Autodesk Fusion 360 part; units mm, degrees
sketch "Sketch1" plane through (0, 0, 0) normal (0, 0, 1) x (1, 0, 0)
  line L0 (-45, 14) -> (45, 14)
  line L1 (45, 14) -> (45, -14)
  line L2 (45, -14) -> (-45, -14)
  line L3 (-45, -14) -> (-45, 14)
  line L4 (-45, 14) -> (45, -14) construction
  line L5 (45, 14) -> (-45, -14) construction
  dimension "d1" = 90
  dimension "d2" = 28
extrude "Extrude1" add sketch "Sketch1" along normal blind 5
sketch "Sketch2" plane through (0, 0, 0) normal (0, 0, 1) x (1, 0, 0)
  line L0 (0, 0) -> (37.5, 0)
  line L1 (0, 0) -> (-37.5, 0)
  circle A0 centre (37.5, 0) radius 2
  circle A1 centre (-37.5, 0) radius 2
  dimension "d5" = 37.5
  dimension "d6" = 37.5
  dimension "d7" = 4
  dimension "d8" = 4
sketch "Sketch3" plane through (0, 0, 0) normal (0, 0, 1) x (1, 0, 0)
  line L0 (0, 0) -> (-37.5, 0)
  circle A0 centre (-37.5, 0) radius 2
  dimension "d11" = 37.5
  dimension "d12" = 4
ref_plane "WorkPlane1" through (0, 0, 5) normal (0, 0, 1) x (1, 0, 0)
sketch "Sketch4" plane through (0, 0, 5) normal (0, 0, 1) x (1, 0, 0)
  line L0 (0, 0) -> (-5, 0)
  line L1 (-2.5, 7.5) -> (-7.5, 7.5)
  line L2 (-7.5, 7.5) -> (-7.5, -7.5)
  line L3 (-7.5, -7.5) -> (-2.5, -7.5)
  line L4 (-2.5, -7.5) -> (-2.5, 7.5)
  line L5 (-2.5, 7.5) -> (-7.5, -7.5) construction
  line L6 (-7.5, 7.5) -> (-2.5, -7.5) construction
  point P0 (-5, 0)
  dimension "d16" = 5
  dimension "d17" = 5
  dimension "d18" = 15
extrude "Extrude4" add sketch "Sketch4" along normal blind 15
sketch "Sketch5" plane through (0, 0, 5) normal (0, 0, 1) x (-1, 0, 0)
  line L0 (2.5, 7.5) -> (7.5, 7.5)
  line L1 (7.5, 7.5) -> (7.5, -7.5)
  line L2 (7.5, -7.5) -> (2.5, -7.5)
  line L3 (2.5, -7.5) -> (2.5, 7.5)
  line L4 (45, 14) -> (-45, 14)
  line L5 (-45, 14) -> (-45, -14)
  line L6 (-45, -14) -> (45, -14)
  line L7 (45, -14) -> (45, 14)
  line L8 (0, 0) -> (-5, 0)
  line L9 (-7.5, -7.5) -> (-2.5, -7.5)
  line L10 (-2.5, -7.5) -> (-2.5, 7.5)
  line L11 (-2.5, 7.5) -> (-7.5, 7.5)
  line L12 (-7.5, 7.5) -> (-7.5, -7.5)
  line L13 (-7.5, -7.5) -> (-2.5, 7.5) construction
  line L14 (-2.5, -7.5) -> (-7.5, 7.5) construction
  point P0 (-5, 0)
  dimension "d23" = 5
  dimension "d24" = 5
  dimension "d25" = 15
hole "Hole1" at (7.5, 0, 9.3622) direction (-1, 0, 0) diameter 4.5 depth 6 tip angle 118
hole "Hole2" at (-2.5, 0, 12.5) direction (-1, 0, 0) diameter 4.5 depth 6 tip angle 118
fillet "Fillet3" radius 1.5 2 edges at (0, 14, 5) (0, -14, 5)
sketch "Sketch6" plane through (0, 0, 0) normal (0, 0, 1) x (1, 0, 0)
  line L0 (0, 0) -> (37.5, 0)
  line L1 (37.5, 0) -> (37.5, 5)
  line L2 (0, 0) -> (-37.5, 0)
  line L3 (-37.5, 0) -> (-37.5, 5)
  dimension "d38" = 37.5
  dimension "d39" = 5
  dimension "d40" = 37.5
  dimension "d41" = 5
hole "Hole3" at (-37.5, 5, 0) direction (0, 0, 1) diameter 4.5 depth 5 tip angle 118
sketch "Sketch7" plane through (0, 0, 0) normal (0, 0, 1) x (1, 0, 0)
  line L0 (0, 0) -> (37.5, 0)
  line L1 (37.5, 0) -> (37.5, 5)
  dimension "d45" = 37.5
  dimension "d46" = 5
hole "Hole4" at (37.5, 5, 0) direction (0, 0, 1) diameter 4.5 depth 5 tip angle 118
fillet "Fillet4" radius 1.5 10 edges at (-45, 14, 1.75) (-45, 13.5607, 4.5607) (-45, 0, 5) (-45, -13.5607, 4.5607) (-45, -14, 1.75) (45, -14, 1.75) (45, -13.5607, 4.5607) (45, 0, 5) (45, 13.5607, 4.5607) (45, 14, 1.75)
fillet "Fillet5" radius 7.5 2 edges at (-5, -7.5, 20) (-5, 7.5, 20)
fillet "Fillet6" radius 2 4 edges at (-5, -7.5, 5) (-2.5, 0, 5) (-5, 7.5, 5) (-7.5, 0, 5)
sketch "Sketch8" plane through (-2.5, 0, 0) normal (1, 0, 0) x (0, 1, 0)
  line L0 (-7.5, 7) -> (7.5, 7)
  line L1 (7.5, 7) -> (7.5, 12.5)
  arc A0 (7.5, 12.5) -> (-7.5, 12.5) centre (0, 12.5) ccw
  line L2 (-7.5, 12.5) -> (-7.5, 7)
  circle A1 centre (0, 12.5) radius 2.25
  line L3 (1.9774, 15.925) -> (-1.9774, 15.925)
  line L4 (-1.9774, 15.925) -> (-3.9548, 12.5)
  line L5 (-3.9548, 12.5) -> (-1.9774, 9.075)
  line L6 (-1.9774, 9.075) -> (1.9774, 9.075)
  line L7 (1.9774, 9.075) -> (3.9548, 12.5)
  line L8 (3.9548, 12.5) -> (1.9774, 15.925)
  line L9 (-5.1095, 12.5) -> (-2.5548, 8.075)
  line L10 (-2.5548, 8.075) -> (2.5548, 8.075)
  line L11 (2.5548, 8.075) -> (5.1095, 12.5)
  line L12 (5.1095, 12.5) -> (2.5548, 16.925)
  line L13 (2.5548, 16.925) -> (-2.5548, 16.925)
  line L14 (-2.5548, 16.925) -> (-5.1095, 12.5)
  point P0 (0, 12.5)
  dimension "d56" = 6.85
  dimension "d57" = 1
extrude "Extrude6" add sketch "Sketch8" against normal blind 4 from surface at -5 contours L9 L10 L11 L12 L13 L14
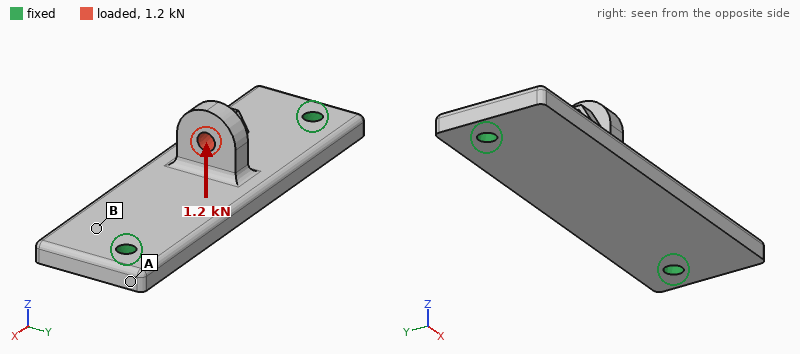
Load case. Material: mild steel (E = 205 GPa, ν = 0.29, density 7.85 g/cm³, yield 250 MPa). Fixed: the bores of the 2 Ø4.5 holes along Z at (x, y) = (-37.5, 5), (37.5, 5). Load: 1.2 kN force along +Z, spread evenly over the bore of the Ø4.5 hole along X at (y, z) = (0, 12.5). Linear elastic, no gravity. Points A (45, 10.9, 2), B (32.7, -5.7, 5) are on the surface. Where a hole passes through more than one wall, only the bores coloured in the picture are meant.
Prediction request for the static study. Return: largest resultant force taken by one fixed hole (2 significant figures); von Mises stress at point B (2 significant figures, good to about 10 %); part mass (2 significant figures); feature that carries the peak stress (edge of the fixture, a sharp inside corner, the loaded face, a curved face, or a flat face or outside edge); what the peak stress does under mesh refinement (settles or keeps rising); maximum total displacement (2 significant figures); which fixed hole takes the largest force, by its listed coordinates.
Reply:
710 N
39 MPa
110 g
edge of the fixture
keeps rising
57 µm
(-37.5, 5)
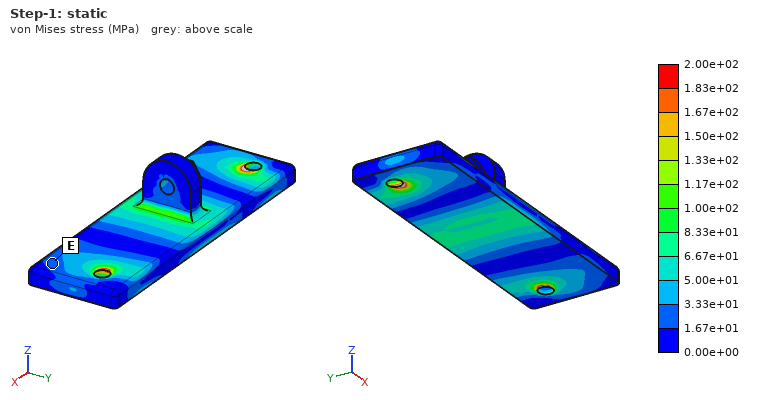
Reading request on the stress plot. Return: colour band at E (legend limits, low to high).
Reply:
1.67e+01 to 3.33e+01 MPa
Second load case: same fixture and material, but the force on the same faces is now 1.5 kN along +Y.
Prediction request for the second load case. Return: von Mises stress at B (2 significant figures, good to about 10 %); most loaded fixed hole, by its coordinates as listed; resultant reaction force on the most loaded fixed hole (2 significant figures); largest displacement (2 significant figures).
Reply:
39 MPa
(-37.5, 5)
1.0 kN
66 µm
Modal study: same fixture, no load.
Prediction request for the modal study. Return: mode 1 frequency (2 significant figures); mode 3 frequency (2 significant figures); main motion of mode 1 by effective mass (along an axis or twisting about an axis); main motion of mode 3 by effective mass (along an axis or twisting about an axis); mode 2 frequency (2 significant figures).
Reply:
3700 Hz
9100 Hz
along Z
twisting about Y
5900 Hz
